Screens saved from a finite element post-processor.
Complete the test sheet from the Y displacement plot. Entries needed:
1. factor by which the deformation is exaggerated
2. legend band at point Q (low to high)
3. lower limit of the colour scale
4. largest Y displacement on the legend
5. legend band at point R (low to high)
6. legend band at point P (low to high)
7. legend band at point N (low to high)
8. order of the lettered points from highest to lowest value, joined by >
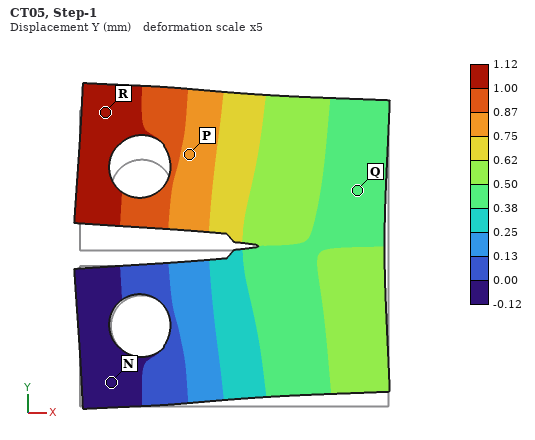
5
0.38 to 0.50 mm
-0.12 mm
1.12 mm
1.00 to 1.12 mm
0.75 to 0.87 mm
-0.12 to 0.00 mm
R > P > Q > N
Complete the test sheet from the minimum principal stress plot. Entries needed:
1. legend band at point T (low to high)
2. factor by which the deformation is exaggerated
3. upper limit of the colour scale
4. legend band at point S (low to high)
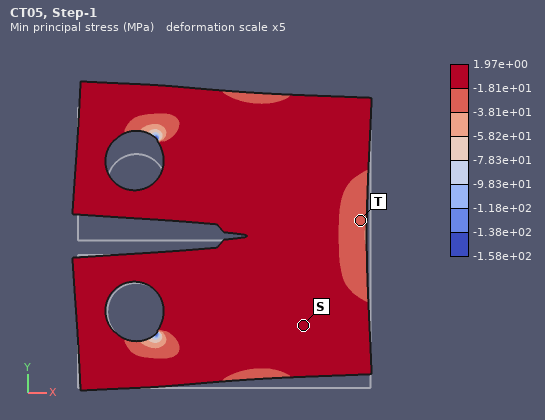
-3.81e+01 to -1.81e+01 MPa
5
1.97e+00 MPa
-1.81e+01 to 1.97e+00 MPa
